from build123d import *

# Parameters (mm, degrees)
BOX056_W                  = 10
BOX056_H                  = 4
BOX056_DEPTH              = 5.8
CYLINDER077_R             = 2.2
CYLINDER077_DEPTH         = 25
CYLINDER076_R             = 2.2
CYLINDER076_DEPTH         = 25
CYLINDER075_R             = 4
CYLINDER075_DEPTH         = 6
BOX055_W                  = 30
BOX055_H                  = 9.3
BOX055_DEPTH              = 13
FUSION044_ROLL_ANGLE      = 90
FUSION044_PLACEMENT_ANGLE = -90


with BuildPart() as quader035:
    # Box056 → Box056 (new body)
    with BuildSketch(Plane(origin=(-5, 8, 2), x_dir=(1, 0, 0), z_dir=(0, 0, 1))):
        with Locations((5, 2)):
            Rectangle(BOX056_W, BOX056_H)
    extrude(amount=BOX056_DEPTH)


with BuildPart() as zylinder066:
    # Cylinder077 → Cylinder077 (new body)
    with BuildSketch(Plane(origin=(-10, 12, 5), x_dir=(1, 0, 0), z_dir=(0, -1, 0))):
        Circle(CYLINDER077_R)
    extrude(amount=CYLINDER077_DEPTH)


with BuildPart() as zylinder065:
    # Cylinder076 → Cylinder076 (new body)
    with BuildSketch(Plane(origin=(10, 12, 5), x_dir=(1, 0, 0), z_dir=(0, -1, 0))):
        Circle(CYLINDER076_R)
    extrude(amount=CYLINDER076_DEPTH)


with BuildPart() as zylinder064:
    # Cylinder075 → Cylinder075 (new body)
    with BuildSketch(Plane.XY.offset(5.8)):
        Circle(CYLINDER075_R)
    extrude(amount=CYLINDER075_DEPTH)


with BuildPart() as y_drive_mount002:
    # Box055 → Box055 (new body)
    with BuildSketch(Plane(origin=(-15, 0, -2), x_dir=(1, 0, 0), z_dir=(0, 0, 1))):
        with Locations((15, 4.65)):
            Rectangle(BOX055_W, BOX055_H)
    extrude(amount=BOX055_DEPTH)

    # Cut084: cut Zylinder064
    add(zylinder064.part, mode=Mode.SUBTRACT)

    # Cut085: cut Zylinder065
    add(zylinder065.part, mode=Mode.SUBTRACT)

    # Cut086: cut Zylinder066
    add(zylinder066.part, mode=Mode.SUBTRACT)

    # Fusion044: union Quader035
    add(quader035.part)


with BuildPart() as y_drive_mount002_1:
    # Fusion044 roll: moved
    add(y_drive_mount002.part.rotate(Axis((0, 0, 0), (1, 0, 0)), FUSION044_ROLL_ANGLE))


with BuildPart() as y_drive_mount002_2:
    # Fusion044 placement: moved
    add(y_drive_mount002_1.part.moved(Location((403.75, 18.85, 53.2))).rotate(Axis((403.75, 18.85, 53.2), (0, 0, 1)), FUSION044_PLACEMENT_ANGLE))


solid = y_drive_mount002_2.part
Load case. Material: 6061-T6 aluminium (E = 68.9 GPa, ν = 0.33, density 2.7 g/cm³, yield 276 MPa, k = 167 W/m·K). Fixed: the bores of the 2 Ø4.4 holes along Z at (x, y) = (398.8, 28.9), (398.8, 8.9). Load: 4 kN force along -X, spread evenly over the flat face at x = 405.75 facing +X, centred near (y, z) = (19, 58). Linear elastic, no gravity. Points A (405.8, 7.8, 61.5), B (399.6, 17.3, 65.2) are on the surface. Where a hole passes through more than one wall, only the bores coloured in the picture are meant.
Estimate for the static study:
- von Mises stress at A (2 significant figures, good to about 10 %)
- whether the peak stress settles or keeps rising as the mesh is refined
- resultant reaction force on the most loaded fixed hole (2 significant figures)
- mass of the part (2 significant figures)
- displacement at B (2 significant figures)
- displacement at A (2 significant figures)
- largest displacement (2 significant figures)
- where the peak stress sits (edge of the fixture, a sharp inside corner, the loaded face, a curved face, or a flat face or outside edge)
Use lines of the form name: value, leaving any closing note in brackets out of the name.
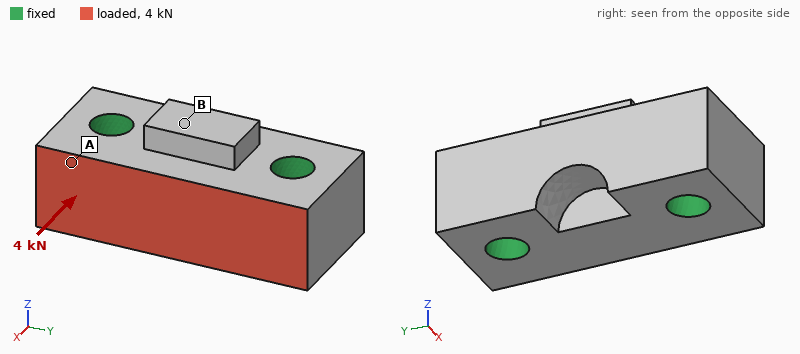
von Mises stress at A: 19 MPa
whether the peak stress settles or keeps rising as the mesh is refined: keeps rising
resultant reaction force on the most loaded fixed hole: 2.0 kN
mass of the part: 9.1 g
displacement at B: 2.6 µm
displacement at A: 1.3 µm
largest displacement: 3.8 µm
where the peak stress sits: edge of the fixture
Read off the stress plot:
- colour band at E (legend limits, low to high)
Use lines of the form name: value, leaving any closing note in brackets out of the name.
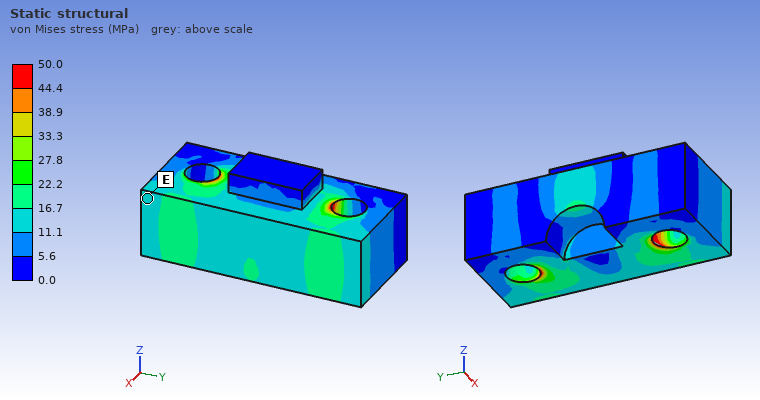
colour band at E: 11.1 to 16.7 MPa
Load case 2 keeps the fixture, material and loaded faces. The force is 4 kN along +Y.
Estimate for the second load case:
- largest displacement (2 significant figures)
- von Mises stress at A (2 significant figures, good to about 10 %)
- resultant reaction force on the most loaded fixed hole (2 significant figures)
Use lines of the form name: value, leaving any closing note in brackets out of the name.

largest displacement: 7.5 µm
von Mises stress at A: 31 MPa
resultant reaction force on the most loaded fixed hole: 2.2 kN
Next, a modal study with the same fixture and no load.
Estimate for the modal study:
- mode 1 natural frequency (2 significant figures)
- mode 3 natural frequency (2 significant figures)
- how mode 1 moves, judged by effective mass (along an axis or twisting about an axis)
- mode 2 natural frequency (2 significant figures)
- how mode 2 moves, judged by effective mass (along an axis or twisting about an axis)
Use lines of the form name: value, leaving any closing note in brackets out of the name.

mode 1 natural frequency: 59 kHz
mode 3 natural frequency: 75 kHz
how mode 1 moves, judged by effective mass: along X
mode 2 natural frequency: 64 kHz
how mode 2 moves, judged by effective mass: along Z
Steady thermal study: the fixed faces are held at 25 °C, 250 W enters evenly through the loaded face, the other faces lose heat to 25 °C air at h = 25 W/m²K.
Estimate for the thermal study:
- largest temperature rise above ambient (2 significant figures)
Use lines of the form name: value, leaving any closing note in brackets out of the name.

largest temperature rise above ambient: 46 K
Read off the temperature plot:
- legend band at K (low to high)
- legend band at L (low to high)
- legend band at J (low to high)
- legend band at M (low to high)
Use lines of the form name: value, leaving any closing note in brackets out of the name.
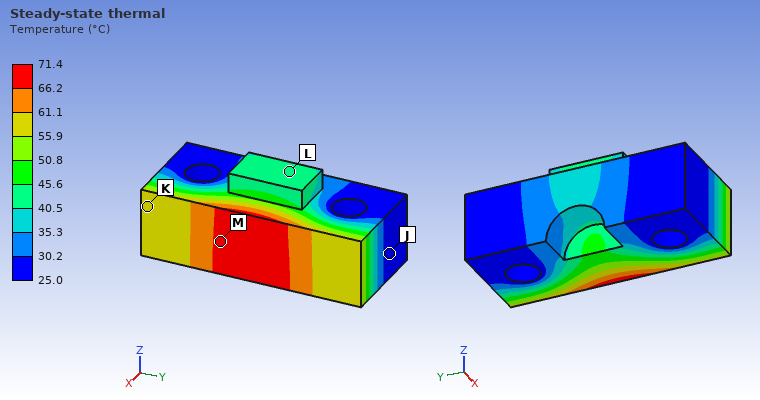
legend band at K: 55.9 to 61.1 °C
legend band at L: 40.5 to 45.6 °C
legend band at J: 25.0 to 30.2 °C
legend band at M: 66.2 to 71.4 °C
